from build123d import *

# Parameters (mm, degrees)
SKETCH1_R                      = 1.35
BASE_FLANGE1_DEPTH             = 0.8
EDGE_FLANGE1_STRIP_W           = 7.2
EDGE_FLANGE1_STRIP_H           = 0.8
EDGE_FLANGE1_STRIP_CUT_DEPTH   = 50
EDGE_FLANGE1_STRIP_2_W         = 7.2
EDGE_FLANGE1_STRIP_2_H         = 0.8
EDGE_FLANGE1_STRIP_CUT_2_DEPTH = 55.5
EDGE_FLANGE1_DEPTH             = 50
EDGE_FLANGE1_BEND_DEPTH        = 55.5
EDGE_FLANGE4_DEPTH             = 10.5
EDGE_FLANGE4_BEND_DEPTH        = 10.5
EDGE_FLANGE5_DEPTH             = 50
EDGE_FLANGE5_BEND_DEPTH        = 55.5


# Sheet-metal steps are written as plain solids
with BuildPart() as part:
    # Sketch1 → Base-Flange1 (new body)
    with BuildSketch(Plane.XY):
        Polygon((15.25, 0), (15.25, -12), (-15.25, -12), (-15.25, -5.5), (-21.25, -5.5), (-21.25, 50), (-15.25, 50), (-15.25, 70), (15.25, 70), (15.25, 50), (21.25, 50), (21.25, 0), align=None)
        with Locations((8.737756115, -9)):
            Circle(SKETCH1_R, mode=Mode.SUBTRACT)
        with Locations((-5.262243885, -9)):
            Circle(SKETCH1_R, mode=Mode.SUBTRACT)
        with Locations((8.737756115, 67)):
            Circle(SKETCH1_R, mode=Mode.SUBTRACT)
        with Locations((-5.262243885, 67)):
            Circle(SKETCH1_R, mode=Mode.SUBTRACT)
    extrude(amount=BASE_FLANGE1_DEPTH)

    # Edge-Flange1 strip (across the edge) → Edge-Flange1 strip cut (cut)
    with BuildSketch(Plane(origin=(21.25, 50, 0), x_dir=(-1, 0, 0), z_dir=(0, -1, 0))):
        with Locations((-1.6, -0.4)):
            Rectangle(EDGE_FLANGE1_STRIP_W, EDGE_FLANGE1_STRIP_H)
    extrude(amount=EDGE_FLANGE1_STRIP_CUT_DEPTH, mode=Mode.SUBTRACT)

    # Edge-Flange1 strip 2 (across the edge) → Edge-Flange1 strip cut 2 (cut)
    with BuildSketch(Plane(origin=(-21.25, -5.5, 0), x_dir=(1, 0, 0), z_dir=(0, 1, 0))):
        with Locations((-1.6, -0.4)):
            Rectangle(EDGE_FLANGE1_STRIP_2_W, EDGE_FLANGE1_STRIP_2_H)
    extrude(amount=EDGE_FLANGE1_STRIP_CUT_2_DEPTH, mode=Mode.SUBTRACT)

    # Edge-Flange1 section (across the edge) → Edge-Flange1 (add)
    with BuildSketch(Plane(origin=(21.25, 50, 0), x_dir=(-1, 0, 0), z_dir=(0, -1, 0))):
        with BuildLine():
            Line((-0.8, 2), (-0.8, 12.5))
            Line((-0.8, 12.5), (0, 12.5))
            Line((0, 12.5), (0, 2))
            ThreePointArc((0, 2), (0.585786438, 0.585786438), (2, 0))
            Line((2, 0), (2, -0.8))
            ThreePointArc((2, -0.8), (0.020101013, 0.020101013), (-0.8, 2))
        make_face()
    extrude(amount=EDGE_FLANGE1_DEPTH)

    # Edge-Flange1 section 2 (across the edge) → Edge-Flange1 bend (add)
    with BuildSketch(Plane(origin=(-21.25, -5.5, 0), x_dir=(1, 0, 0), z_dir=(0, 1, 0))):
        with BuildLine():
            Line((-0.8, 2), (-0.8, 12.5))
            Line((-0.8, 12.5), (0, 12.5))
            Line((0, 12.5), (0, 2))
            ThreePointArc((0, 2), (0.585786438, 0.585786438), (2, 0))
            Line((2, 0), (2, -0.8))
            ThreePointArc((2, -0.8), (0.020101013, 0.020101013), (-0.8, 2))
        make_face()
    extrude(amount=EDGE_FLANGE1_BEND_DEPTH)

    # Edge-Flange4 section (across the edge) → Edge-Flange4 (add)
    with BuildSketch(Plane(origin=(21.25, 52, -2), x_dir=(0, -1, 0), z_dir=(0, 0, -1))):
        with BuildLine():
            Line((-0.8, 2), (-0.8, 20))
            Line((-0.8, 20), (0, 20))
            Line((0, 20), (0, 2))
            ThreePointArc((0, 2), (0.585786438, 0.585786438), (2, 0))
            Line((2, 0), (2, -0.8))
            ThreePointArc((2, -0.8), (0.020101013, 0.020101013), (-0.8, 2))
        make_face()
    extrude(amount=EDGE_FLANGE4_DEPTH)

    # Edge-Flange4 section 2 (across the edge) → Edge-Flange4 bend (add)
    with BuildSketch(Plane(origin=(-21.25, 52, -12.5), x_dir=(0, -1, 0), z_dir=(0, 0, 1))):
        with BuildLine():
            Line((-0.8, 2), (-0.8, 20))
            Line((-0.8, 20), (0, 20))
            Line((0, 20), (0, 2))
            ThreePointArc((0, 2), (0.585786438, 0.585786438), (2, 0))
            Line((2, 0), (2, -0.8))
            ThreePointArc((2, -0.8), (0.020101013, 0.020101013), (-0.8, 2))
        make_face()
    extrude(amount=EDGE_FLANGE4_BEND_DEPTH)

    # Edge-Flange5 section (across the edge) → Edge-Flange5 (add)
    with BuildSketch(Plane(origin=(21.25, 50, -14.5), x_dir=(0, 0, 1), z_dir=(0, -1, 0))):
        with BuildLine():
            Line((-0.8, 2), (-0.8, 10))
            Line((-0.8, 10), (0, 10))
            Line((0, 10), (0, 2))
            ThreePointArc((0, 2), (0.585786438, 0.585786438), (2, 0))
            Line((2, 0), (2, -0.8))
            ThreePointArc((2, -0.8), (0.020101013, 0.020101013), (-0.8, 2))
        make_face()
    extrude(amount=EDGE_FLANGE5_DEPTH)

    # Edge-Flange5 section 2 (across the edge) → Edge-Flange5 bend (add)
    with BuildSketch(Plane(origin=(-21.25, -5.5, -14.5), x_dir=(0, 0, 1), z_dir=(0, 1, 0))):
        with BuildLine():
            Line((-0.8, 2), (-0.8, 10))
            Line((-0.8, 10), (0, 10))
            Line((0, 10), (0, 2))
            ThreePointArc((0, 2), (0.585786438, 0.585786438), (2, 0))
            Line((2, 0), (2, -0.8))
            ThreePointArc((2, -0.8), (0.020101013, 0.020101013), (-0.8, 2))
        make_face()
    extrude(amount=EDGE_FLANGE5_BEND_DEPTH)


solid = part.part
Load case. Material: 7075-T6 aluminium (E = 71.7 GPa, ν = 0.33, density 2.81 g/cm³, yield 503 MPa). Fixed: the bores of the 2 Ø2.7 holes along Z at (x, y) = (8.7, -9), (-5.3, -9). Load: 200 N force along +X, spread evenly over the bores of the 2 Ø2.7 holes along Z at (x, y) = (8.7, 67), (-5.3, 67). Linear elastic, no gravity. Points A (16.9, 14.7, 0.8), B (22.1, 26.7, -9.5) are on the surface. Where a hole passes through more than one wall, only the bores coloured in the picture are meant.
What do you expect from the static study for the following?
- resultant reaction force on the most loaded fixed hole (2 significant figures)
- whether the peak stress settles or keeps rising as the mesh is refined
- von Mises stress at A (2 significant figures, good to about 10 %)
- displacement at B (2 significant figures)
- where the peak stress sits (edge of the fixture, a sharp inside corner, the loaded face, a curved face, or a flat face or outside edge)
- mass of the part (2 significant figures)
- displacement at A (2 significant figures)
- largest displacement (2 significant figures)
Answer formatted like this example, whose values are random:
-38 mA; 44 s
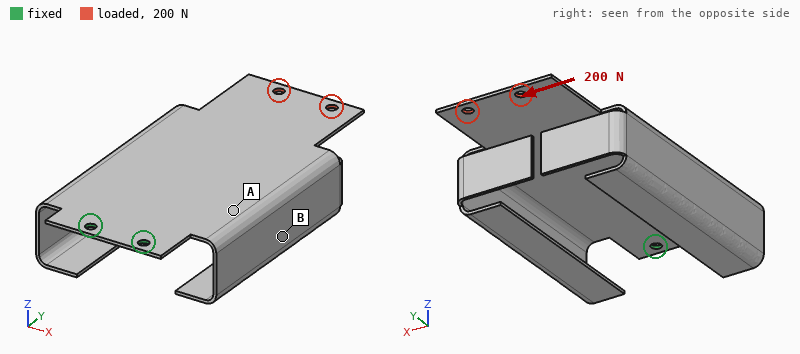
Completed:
960 N; keeps rising; 28 MPa; 0.14 mm; edge of the fixture; 14 g; 0.090 mm; 0.29 mm
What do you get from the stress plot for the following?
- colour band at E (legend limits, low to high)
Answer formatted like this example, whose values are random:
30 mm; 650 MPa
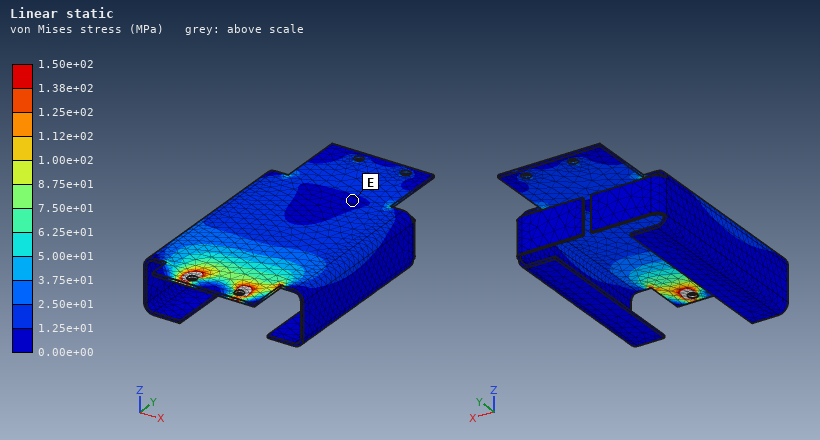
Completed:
0.00e+00 to 1.25e+01 MPa
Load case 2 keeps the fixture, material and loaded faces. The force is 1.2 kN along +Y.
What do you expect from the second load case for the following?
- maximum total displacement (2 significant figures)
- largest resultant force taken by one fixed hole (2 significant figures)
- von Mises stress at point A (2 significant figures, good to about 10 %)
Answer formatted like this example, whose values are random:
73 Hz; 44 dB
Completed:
91 µm; 600 N; 35 MPa
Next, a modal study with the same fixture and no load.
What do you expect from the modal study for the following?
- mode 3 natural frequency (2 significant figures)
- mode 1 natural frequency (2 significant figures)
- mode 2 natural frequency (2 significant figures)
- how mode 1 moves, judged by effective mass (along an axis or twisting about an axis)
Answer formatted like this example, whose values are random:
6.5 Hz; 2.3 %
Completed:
600 Hz; 100 Hz; 240 Hz; along Z
